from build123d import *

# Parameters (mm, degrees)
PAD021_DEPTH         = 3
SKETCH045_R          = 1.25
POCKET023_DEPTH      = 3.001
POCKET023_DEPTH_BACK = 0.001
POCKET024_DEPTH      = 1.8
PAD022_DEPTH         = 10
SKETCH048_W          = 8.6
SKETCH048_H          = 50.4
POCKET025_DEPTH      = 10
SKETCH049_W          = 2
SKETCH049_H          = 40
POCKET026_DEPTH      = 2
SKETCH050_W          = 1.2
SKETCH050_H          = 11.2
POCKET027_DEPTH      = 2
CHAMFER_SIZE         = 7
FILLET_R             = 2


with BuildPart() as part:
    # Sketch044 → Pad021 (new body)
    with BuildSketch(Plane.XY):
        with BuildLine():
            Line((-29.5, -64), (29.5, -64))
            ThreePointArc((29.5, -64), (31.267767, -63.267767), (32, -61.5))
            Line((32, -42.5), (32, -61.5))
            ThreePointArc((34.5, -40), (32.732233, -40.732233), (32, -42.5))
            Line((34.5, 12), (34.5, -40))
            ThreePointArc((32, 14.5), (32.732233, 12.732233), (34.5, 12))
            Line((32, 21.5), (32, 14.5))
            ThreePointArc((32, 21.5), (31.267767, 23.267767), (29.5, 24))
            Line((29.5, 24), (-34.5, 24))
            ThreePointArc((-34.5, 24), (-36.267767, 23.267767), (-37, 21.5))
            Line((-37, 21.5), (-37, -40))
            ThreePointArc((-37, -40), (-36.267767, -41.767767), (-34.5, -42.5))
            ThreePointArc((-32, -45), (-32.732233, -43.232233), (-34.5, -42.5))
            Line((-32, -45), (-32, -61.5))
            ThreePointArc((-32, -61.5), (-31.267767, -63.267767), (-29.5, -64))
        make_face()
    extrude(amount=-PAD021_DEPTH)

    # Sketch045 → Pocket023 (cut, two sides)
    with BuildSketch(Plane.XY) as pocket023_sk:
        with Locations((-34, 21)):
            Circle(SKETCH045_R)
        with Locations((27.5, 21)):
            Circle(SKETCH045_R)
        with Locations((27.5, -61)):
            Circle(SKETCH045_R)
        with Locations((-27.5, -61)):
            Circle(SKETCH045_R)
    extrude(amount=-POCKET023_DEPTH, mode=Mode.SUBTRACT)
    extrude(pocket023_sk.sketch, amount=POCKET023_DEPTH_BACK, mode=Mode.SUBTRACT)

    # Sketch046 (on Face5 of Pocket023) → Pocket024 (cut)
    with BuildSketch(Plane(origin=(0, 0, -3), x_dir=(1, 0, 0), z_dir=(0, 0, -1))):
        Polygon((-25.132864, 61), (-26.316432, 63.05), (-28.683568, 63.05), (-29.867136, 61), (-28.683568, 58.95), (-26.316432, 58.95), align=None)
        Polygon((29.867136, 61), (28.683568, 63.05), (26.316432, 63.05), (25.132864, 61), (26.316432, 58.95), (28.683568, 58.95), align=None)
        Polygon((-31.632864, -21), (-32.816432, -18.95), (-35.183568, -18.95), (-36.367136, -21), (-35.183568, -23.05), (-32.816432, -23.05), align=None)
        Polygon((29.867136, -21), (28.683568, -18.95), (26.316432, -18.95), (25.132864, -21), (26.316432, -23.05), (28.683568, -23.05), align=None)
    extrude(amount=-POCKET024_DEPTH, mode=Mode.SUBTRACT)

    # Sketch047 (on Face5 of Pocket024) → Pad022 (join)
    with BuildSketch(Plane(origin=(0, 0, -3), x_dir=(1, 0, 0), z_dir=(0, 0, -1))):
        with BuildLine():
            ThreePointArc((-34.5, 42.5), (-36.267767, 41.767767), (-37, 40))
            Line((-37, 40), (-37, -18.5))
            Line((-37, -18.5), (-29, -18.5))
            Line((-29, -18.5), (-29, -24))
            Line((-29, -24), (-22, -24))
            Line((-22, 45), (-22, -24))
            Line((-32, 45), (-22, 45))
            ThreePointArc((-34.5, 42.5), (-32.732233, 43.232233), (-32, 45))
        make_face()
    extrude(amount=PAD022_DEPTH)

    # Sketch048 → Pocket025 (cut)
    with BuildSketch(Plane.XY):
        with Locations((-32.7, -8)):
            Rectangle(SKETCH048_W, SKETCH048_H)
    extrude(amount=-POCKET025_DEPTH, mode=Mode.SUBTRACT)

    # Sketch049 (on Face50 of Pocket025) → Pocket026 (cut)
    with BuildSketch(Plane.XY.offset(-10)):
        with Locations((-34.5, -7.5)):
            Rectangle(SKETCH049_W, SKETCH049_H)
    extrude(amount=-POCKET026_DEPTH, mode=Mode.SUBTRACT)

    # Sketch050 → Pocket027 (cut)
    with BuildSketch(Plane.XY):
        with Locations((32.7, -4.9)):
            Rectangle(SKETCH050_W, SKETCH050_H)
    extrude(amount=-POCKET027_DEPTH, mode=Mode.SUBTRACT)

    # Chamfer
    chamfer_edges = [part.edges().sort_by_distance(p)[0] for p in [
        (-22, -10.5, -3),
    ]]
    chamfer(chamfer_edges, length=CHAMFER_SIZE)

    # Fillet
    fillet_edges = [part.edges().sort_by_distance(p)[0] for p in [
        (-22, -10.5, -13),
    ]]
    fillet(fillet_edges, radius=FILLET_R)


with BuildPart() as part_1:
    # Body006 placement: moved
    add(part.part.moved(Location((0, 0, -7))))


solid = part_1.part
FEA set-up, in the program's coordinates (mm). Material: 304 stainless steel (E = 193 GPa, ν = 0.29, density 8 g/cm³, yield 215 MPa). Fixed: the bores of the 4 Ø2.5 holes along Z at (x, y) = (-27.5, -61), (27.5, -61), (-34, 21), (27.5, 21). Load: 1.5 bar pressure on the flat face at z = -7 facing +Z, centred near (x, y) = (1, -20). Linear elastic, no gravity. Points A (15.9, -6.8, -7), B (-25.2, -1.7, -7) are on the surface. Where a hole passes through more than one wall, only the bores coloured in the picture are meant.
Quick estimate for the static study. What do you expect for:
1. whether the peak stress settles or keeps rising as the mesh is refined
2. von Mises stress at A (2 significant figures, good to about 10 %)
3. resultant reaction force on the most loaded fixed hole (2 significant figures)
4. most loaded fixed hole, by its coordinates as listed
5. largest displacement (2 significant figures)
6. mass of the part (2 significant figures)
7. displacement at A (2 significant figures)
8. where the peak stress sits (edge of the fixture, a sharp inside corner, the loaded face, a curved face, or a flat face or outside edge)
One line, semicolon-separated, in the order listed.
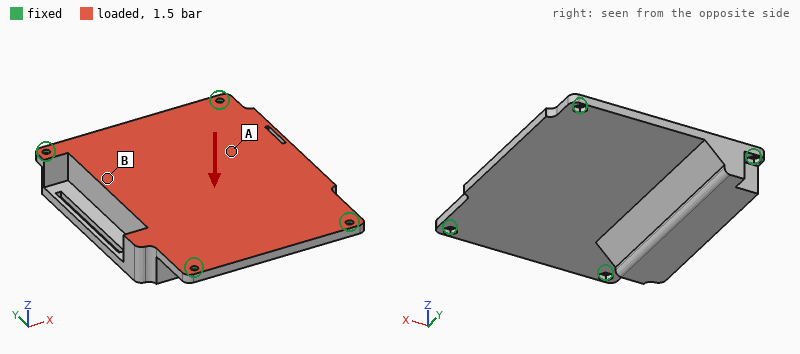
keeps rising; 25 MPa; 580 N; (27.5, 21); 76 µm; 200 g; 64 µm; edge of the fixture
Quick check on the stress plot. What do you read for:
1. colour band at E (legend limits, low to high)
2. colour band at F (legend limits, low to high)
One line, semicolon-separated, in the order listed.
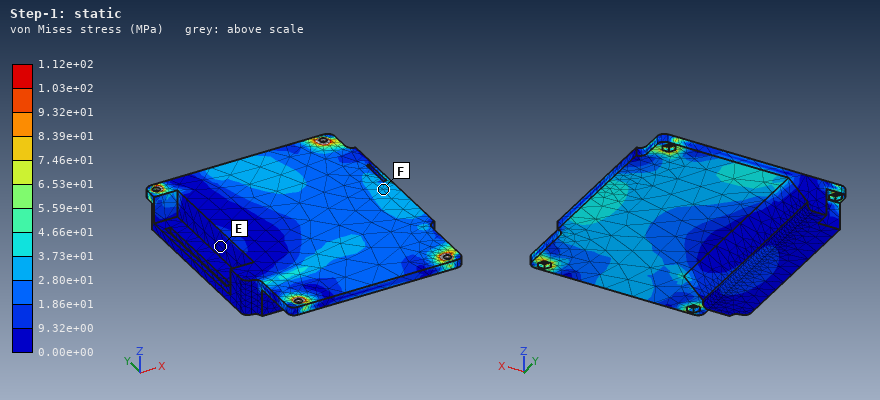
0.00e+00 to 9.32e+00 MPa; 2.80e+01 to 3.73e+01 MPa
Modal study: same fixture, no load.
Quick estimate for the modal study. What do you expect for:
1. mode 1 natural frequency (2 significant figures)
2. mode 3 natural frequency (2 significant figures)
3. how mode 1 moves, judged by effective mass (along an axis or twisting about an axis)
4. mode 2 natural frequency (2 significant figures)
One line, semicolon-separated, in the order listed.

1700 Hz; 3200 Hz; along Z; 2700 Hz
